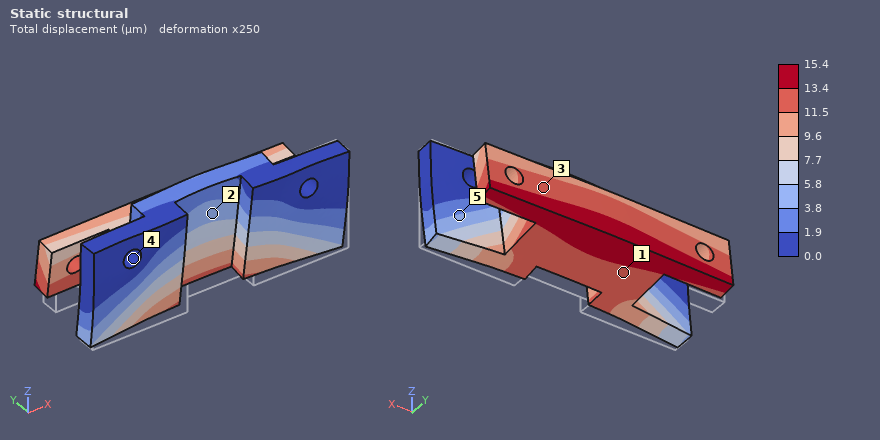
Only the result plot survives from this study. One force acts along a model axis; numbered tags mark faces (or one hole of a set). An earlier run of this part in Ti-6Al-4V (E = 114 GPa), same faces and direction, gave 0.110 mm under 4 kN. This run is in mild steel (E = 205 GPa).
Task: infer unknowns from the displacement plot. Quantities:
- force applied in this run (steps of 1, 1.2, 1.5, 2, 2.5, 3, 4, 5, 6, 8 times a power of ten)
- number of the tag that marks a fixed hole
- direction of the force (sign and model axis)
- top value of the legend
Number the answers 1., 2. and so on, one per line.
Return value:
1. 1 kN
2. 4
3. +Y
4. 15.4 µm
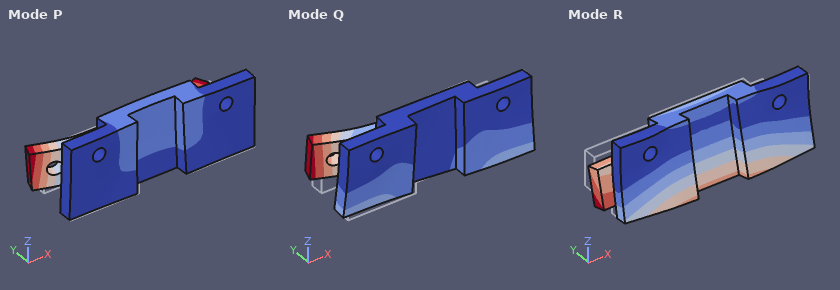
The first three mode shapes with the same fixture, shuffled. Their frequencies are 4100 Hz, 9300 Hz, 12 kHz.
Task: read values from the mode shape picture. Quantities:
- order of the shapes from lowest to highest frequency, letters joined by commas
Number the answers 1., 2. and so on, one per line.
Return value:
1. R, Q, P
